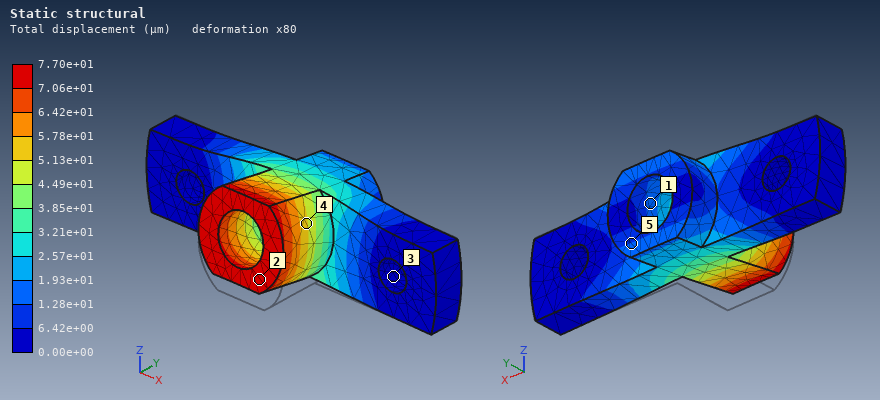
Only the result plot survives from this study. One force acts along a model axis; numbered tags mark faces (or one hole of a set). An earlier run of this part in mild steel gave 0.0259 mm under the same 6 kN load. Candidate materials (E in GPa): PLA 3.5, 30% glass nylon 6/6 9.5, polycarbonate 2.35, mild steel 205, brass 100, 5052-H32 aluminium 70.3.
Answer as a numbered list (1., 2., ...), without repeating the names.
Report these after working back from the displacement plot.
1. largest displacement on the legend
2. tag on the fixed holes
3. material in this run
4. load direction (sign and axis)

1. 7.70e+01 µm
2. 3
3. 5052-H32 aluminium
4. +Z
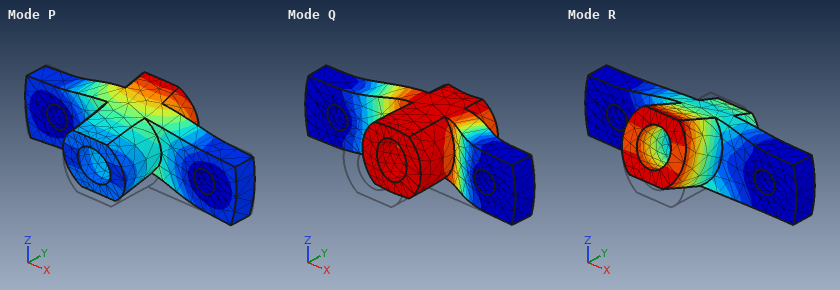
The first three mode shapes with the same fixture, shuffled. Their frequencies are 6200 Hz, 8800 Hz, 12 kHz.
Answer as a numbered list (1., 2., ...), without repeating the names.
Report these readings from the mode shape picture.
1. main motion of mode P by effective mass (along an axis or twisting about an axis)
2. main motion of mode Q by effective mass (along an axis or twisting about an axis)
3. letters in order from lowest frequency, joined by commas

1. along Z
2. along Y
3. R, Q, P
